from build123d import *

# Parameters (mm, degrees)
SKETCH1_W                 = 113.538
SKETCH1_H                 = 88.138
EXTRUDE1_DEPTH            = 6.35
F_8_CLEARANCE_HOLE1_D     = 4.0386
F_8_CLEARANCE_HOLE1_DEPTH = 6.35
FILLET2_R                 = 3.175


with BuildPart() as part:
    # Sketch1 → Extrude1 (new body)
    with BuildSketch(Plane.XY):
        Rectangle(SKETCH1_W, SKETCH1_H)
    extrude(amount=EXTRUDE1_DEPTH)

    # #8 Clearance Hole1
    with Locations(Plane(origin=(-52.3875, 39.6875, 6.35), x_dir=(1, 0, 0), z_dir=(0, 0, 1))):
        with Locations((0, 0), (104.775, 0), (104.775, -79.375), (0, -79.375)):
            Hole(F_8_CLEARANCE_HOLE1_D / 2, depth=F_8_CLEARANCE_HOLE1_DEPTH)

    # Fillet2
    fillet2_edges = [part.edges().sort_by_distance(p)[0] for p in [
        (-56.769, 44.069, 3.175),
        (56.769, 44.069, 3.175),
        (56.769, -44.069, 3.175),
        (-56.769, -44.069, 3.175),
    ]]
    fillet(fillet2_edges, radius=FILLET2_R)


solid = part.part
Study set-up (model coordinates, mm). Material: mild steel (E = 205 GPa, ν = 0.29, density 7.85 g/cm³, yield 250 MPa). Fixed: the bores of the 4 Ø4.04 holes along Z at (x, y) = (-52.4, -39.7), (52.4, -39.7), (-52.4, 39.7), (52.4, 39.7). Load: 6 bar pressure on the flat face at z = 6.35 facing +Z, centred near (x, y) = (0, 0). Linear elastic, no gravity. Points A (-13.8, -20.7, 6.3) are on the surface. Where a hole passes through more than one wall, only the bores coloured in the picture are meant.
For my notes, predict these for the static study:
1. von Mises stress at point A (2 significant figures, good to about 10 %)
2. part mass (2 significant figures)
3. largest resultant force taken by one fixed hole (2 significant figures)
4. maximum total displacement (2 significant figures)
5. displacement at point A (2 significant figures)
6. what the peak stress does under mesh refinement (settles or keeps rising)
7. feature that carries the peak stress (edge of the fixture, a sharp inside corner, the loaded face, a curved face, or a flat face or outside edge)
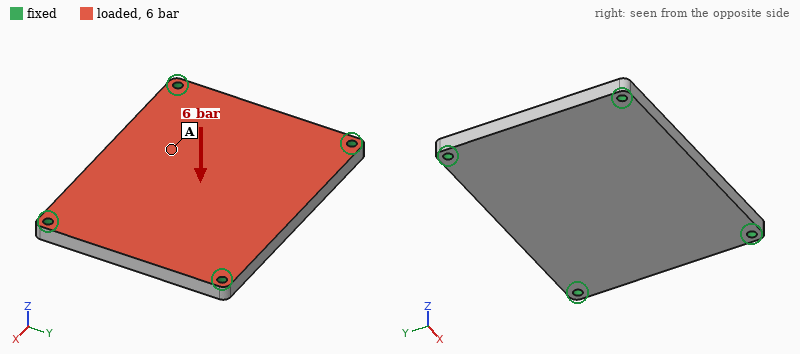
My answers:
45 MPa
500 g
1.5 kN
95 µm
82 µm
keeps rising
edge of the fixture
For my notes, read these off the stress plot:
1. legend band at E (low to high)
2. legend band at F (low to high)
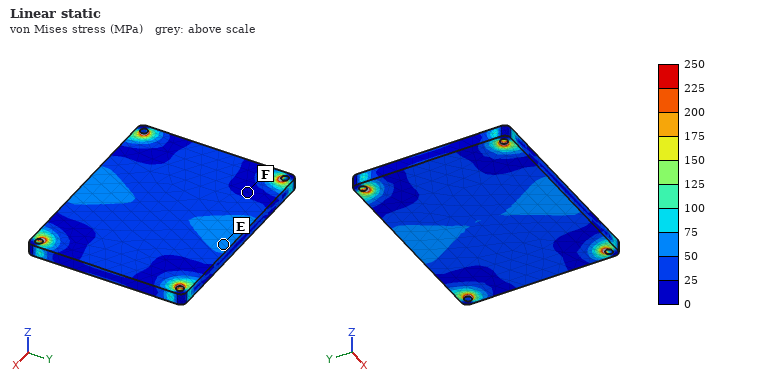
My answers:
50 to 75 MPa
0 to 25 MPa
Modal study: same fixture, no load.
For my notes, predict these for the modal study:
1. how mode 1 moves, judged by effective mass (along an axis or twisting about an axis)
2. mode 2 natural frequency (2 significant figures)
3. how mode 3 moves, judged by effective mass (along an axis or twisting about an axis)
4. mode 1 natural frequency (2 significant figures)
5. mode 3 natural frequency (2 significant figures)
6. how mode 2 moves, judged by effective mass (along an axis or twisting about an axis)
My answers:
along Z
3600 Hz
twisting about Y
2100 Hz
4600 Hz
twisting about X
